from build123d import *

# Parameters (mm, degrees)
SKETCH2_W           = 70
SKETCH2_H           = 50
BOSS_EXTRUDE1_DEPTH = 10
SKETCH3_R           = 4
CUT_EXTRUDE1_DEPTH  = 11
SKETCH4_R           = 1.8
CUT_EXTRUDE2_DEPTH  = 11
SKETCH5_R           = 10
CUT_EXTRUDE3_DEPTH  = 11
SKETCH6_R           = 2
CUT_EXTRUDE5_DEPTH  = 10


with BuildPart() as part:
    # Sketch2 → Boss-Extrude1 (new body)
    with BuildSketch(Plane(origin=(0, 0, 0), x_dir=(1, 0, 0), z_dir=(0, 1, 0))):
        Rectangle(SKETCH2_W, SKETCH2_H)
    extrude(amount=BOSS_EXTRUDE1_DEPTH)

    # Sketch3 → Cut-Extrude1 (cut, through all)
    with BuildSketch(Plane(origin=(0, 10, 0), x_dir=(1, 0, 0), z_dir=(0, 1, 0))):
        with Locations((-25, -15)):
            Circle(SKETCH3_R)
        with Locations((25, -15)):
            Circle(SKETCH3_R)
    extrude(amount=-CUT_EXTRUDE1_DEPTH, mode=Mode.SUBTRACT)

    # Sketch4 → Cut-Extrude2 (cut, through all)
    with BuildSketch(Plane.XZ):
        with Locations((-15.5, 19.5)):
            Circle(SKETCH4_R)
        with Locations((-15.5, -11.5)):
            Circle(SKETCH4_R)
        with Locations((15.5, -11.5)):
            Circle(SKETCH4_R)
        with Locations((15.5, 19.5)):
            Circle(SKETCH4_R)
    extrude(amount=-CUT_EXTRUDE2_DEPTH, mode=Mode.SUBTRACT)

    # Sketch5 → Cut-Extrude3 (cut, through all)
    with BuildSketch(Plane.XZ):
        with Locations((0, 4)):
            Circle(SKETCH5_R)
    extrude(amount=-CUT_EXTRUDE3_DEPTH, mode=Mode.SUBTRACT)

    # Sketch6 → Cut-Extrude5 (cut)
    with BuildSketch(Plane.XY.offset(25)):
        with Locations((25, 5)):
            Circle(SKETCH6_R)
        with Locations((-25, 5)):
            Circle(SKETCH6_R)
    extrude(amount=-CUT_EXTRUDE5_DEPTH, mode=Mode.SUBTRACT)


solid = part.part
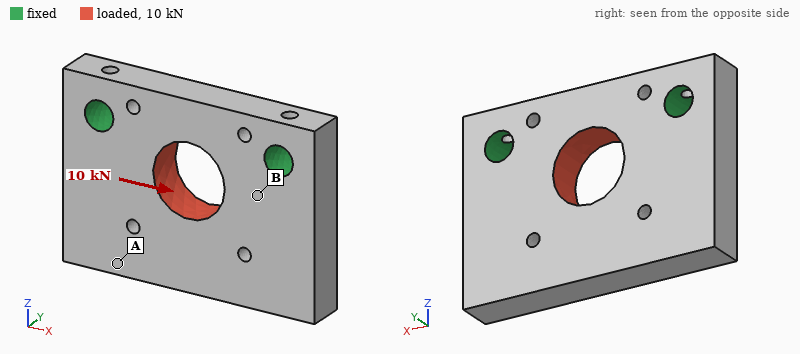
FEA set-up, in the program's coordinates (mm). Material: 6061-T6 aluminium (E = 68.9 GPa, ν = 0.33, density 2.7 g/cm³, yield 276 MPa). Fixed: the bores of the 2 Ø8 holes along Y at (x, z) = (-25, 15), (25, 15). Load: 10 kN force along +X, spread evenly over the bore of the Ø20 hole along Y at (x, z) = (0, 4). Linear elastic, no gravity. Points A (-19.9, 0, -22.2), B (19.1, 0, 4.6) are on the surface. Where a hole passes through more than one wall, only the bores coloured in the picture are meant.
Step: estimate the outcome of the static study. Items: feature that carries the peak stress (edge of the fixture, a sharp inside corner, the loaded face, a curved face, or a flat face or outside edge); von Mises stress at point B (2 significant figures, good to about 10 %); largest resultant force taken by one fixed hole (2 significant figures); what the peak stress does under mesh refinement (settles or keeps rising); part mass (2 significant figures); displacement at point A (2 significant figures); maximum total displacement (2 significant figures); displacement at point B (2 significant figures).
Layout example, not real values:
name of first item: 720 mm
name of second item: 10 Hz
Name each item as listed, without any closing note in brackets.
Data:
feature that carries the peak stress: edge of the fixture
von Mises stress at point B: 27 MPa
largest resultant force taken by one fixed hole: 5.2 kN
what the peak stress does under mesh refinement: keeps rising
part mass: 82 g
displacement at point A: 16 µm
maximum total displacement: 18 µm
displacement at point B: 7.4 µm
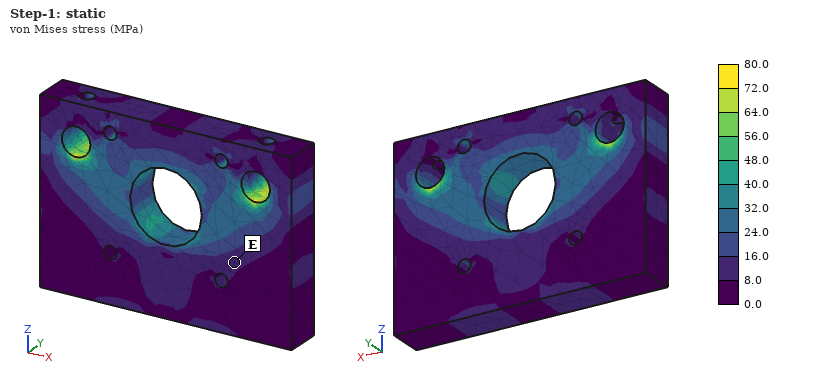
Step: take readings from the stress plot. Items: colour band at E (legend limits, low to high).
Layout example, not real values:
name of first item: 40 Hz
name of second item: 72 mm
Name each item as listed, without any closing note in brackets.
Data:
colour band at E: 8.0 to 16.0 MPa
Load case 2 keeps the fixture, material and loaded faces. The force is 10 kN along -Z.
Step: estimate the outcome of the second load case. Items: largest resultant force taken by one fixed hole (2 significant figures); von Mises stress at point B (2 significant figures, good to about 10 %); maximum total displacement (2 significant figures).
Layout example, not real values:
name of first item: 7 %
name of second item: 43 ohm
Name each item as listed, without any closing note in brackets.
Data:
largest resultant force taken by one fixed hole: 5.1 kN
von Mises stress at point B: 30 MPa
maximum total displacement: 17 µm
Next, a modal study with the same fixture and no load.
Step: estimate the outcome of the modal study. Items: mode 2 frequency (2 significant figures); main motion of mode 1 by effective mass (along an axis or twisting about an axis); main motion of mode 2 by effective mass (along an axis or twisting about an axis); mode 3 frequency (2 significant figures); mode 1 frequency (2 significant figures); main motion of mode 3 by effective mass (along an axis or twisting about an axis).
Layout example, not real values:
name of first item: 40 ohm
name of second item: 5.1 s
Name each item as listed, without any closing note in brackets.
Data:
mode 2 frequency: 7600 Hz
main motion of mode 1 by effective mass: along Y
main motion of mode 2 by effective mass: twisting about Z
mode 3 frequency: 13 kHz
mode 1 frequency: 4400 Hz
main motion of mode 3 by effective mass: along X
